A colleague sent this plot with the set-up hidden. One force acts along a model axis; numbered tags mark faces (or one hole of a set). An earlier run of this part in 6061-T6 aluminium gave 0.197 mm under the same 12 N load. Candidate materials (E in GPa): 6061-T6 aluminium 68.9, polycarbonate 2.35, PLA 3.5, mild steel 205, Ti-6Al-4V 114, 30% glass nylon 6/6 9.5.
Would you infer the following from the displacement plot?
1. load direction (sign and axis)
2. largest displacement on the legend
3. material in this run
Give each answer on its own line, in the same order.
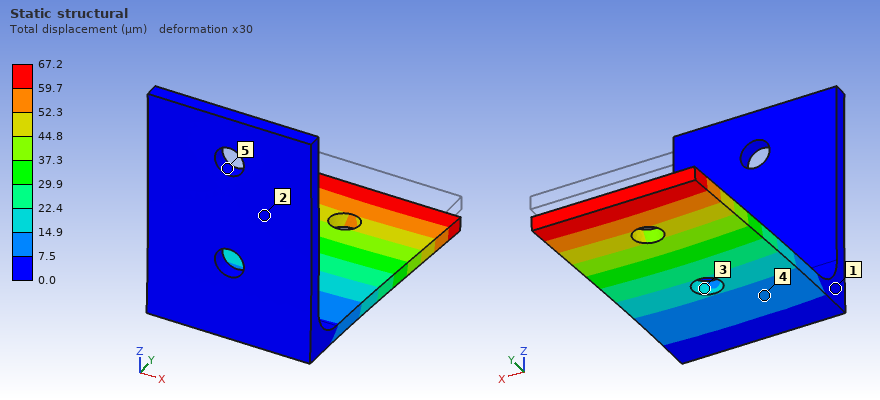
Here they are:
-Z
67.2 µm
mild steel
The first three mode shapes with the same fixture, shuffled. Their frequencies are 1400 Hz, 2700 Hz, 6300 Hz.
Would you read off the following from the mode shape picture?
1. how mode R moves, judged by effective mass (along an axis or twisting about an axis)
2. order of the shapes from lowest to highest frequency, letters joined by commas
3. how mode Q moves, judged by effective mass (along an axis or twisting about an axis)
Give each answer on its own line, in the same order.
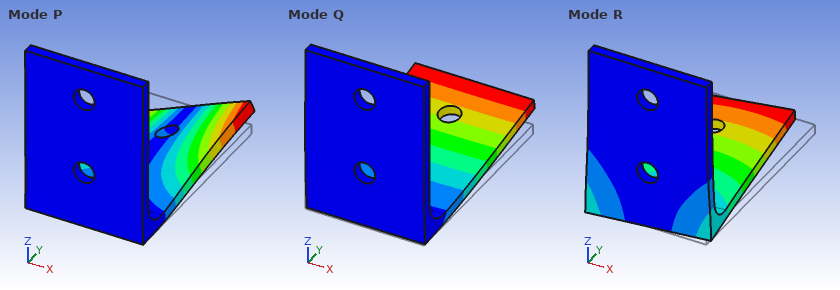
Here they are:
along X
Q, R, P
along Z
